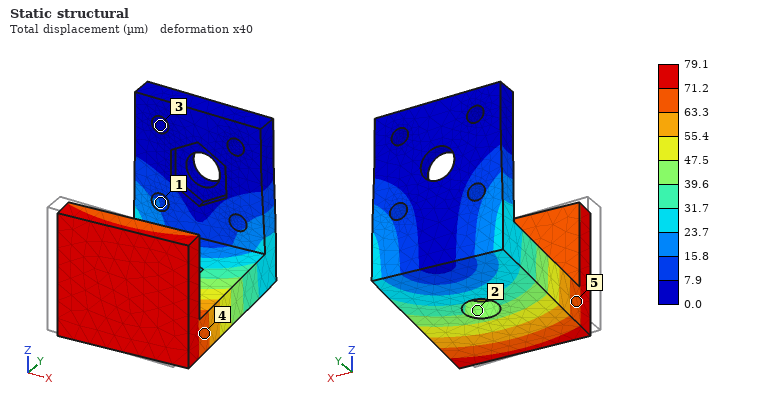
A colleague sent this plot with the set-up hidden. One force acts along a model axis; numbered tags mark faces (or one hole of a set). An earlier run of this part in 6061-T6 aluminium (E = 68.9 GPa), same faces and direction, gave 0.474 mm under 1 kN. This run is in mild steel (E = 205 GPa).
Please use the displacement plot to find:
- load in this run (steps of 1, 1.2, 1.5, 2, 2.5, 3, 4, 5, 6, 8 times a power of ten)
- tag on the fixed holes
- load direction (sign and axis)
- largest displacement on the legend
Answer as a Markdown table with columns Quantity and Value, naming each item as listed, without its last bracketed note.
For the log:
| Quantity | Value |
|---|---|
| load in this run | 500 N |
| tag on the fixed holes | 3 |
| load direction | +X |
| largest displacement on the legend | 79.1 µm |
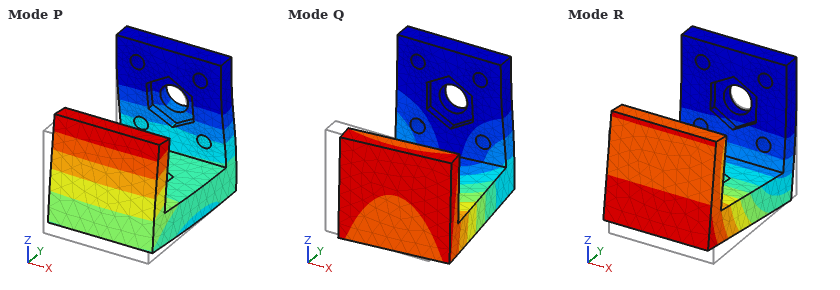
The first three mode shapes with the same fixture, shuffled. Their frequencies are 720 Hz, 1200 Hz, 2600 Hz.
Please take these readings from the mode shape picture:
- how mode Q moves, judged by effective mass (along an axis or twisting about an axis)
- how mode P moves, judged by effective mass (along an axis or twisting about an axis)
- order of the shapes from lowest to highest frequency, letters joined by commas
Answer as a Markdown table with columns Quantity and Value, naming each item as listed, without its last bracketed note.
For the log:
| Quantity | Value |
|---|---|
| how mode Q moves, judged by effective mass | along X |
| how mode P moves, judged by effective mass | along Y |
| order of the shapes from lowest to highest frequency, letters joined by commas | R, Q, P |
